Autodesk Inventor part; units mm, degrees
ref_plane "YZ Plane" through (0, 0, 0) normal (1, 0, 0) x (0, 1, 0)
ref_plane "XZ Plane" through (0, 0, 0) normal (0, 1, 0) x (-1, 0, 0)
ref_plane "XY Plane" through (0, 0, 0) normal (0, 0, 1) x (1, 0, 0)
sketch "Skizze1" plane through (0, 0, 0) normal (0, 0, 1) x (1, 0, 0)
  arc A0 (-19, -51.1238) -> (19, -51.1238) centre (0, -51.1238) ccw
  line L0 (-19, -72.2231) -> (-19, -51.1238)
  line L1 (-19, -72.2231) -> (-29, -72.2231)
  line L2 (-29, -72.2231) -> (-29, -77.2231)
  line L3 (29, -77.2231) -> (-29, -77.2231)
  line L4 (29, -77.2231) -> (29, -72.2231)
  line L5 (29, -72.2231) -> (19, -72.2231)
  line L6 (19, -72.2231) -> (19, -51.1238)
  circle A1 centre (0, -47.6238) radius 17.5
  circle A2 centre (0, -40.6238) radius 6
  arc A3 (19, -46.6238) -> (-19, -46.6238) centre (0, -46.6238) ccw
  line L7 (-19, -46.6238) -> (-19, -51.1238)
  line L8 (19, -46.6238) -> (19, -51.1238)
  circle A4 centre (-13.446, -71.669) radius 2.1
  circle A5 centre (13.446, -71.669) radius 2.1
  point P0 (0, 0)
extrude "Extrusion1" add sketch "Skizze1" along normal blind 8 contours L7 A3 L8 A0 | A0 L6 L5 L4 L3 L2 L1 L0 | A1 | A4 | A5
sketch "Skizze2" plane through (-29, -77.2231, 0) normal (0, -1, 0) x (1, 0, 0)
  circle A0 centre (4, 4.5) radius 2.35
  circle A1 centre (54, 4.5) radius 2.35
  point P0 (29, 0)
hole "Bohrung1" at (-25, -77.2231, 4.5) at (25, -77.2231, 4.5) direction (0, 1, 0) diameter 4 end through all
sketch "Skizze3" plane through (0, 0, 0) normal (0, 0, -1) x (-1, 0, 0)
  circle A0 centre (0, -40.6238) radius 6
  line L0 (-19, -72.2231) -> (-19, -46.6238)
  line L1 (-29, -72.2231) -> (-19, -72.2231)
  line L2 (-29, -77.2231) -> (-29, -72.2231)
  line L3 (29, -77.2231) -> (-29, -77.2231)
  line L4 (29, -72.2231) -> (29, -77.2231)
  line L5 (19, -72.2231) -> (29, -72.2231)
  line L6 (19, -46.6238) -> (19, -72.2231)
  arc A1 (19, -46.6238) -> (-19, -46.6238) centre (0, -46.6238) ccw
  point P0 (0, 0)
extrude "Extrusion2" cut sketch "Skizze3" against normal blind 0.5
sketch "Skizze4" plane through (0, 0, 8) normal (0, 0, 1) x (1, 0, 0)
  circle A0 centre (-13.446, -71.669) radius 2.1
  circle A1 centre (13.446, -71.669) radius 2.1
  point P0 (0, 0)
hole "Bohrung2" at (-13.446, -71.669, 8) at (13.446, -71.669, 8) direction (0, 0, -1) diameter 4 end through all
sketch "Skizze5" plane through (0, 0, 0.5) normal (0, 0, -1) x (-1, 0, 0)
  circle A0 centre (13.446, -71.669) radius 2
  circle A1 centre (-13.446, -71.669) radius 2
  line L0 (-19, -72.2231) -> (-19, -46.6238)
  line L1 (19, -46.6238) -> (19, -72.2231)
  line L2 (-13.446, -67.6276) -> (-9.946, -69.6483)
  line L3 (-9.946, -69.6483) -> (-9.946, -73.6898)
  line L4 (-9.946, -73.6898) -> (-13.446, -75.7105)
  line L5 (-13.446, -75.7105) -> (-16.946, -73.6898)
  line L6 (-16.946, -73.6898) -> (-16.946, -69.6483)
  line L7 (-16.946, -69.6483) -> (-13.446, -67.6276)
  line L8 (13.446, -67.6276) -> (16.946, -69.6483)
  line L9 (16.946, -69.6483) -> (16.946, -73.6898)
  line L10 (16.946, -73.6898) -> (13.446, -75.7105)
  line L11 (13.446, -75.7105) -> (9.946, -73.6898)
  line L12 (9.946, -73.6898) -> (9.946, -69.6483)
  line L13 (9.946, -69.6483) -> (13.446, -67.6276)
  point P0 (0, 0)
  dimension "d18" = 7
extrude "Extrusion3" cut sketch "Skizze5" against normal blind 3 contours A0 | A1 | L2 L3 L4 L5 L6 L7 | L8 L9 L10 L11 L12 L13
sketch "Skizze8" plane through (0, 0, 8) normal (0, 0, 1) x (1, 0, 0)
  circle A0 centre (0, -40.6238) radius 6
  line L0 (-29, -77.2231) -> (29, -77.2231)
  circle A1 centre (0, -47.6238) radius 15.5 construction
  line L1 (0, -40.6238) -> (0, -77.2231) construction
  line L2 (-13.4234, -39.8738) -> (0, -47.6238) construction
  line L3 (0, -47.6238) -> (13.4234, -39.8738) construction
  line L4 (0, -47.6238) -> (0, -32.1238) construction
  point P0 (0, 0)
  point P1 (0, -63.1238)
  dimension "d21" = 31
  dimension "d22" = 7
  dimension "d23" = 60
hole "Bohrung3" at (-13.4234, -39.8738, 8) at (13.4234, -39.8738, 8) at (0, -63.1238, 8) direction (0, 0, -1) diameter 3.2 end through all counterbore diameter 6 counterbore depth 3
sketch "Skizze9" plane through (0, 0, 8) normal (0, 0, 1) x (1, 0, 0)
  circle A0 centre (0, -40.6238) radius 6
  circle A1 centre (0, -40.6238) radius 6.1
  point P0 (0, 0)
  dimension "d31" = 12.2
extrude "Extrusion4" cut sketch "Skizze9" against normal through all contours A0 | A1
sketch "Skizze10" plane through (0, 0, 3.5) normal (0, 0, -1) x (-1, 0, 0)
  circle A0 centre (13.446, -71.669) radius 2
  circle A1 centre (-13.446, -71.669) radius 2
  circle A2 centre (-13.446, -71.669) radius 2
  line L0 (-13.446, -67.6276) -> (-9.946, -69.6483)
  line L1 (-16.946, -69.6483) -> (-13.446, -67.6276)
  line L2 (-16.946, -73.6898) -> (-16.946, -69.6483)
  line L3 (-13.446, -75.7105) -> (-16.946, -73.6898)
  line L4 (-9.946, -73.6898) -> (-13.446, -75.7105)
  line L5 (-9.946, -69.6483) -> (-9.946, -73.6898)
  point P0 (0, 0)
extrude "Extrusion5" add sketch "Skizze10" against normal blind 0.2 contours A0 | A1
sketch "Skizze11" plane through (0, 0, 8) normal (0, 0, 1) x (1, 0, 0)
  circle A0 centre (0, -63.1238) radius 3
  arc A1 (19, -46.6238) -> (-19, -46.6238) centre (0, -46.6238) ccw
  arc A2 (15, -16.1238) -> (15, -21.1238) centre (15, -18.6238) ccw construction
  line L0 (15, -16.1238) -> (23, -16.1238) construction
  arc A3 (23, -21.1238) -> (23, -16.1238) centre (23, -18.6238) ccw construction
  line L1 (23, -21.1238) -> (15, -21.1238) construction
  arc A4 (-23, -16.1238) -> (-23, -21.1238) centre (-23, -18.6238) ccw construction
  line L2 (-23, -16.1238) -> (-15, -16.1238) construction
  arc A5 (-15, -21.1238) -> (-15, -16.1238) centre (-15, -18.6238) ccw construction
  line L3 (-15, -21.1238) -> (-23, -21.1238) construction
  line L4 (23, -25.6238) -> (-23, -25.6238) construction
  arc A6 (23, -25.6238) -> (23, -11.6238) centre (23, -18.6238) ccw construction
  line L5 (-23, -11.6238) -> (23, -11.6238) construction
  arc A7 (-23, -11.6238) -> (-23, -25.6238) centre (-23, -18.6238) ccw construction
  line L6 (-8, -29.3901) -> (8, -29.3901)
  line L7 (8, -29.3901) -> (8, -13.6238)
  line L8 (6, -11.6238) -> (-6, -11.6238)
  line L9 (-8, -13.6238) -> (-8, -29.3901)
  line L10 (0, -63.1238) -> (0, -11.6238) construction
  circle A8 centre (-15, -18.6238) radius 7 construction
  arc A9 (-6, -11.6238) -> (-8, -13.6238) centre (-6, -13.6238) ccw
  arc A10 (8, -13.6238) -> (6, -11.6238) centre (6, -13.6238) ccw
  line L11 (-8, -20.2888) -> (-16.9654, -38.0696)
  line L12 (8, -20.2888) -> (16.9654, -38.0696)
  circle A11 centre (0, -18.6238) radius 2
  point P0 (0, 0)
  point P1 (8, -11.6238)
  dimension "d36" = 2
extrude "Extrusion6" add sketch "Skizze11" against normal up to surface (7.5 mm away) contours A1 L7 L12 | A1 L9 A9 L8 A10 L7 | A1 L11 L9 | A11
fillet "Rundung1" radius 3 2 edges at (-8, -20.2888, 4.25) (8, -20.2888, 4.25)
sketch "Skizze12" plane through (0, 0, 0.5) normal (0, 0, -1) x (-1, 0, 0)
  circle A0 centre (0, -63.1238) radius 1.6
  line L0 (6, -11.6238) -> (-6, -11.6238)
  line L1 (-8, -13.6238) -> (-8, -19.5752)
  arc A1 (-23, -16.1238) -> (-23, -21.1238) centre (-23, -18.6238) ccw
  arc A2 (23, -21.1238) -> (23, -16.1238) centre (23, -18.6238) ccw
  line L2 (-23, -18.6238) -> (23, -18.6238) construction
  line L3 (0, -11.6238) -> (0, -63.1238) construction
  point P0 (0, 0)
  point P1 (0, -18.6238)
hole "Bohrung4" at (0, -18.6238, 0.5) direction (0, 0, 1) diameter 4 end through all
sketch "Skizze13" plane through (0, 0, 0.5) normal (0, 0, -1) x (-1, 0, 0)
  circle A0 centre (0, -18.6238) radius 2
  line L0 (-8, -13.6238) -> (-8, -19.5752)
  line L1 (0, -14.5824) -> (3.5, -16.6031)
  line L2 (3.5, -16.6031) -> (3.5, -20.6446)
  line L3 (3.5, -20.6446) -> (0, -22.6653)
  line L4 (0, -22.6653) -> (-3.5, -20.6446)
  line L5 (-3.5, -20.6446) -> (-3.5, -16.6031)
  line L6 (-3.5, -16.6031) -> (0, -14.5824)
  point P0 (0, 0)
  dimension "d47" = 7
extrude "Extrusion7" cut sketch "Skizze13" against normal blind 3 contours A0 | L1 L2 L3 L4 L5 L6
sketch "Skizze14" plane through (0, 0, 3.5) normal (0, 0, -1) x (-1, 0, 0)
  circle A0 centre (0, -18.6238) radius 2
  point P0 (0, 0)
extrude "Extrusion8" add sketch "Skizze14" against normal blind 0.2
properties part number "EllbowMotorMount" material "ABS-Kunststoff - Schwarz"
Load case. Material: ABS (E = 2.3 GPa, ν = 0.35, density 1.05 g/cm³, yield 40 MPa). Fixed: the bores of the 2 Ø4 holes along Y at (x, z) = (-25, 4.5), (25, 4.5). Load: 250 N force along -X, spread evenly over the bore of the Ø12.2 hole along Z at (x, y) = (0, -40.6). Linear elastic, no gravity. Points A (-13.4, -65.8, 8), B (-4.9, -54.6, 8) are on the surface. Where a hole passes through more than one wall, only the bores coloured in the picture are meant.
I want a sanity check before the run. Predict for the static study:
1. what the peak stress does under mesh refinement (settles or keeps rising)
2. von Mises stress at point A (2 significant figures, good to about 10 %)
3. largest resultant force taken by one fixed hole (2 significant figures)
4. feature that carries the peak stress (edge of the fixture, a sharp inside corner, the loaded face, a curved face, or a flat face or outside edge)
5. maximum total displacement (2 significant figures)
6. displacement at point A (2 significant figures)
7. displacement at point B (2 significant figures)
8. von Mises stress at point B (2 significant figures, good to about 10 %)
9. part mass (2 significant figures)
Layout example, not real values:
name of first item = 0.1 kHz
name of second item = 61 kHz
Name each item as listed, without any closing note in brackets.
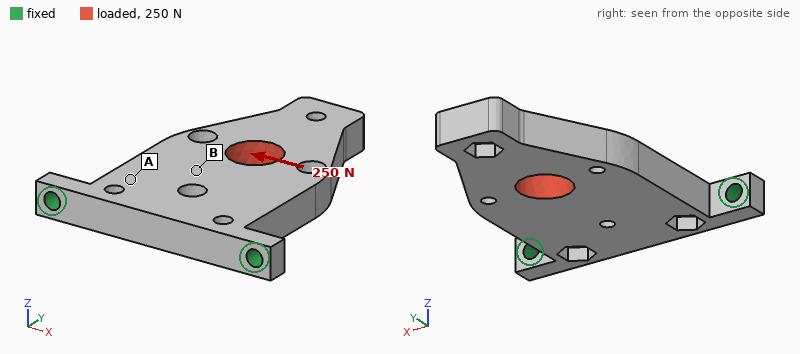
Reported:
what the peak stress does under mesh refinement = keeps rising
von Mises stress at point A = 4.2 MPa
largest resultant force taken by one fixed hole = 240 N
feature that carries the peak stress = edge of the fixture
maximum total displacement = 0.41 mm
displacement at point A = 0.084 mm
displacement at point B = 0.13 mm
von Mises stress at point B = 2.2 MPa
part mass = 15 g
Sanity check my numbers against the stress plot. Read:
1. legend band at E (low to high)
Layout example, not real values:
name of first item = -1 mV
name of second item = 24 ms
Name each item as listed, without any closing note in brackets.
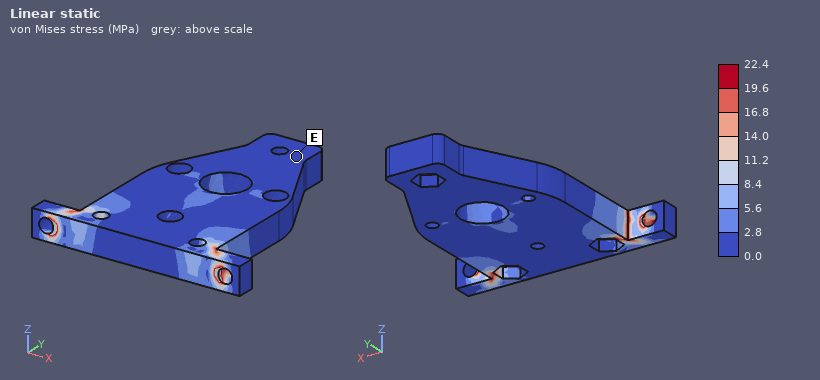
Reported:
legend band at E = 0.0 to 2.8 MPa
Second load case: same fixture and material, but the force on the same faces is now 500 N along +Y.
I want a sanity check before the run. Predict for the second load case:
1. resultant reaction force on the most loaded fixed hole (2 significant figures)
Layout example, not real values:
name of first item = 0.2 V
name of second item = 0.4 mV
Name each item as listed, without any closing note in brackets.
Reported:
resultant reaction force on the most loaded fixed hole = 270 N
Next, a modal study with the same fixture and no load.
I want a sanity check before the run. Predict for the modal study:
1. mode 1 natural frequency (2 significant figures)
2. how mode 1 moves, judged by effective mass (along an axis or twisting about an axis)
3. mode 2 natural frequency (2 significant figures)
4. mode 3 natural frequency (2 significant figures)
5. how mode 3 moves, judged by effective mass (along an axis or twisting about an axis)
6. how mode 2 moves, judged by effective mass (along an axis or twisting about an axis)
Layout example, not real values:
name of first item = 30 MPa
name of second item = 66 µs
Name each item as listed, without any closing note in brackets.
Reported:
mode 1 natural frequency = 260 Hz
how mode 1 moves, judged by effective mass = along Z
mode 2 natural frequency = 1500 Hz
mode 3 natural frequency = 1800 Hz
how mode 3 moves, judged by effective mass = twisting about Y
how mode 2 moves, judged by effective mass = along X
